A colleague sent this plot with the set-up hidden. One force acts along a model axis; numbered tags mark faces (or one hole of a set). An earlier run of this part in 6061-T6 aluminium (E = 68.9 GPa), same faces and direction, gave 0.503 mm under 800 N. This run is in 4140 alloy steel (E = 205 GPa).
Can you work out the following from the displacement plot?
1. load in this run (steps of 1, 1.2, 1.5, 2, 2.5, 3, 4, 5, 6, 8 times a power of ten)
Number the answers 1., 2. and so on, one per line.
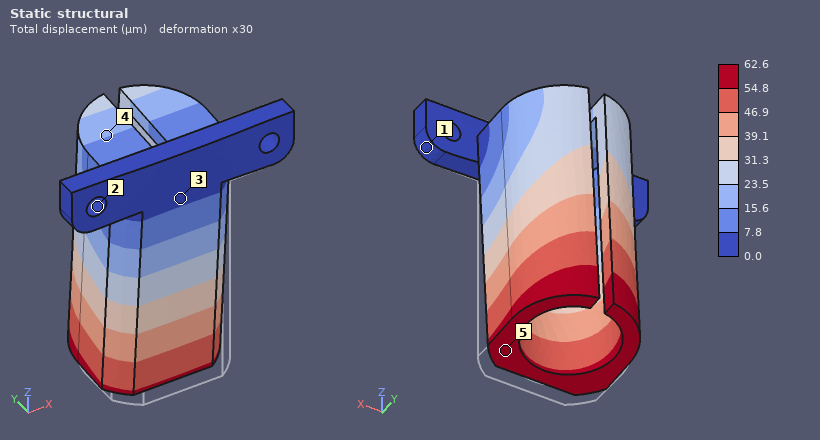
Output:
1. 300 N
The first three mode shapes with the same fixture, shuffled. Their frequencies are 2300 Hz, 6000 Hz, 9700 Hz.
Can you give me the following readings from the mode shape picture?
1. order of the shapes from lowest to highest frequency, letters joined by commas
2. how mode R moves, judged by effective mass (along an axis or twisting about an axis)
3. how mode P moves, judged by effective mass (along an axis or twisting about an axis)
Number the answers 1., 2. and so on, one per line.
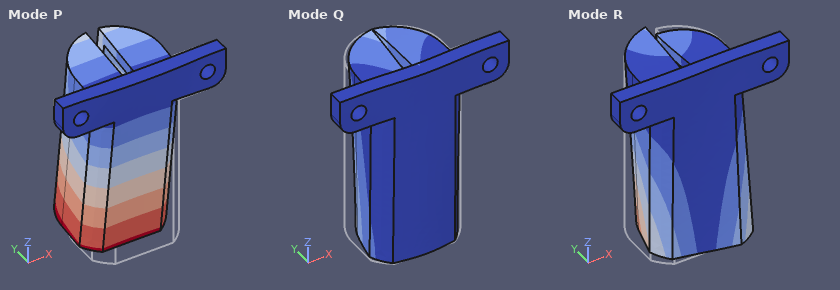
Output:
1. P, R, Q
2. along X
3. along Y
